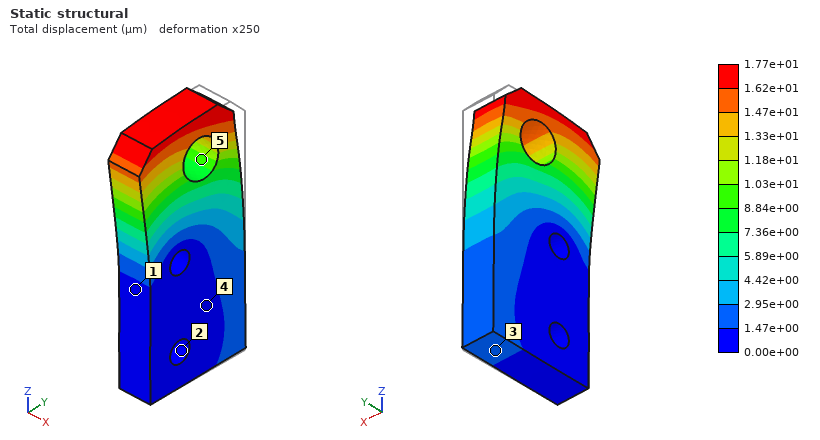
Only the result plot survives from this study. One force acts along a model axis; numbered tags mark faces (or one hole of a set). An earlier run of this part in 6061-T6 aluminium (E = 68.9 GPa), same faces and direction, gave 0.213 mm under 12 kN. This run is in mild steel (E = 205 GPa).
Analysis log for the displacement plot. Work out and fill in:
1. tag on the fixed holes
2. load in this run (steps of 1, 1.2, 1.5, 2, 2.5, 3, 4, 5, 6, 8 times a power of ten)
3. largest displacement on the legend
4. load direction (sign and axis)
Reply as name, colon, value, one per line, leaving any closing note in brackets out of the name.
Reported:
tag on the fixed holes: 2
load in this run: 3 kN
largest displacement on the legend: 1.77e+01 µm
load direction: -Y
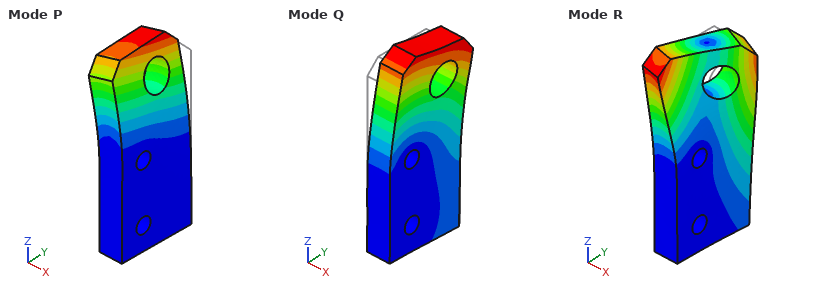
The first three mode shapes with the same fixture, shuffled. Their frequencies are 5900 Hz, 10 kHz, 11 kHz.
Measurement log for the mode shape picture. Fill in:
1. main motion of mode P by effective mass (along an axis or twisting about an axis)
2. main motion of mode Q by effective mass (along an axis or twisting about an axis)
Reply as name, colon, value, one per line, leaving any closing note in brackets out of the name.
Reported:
main motion of mode P by effective mass: along X
main motion of mode Q by effective mass: along Y
